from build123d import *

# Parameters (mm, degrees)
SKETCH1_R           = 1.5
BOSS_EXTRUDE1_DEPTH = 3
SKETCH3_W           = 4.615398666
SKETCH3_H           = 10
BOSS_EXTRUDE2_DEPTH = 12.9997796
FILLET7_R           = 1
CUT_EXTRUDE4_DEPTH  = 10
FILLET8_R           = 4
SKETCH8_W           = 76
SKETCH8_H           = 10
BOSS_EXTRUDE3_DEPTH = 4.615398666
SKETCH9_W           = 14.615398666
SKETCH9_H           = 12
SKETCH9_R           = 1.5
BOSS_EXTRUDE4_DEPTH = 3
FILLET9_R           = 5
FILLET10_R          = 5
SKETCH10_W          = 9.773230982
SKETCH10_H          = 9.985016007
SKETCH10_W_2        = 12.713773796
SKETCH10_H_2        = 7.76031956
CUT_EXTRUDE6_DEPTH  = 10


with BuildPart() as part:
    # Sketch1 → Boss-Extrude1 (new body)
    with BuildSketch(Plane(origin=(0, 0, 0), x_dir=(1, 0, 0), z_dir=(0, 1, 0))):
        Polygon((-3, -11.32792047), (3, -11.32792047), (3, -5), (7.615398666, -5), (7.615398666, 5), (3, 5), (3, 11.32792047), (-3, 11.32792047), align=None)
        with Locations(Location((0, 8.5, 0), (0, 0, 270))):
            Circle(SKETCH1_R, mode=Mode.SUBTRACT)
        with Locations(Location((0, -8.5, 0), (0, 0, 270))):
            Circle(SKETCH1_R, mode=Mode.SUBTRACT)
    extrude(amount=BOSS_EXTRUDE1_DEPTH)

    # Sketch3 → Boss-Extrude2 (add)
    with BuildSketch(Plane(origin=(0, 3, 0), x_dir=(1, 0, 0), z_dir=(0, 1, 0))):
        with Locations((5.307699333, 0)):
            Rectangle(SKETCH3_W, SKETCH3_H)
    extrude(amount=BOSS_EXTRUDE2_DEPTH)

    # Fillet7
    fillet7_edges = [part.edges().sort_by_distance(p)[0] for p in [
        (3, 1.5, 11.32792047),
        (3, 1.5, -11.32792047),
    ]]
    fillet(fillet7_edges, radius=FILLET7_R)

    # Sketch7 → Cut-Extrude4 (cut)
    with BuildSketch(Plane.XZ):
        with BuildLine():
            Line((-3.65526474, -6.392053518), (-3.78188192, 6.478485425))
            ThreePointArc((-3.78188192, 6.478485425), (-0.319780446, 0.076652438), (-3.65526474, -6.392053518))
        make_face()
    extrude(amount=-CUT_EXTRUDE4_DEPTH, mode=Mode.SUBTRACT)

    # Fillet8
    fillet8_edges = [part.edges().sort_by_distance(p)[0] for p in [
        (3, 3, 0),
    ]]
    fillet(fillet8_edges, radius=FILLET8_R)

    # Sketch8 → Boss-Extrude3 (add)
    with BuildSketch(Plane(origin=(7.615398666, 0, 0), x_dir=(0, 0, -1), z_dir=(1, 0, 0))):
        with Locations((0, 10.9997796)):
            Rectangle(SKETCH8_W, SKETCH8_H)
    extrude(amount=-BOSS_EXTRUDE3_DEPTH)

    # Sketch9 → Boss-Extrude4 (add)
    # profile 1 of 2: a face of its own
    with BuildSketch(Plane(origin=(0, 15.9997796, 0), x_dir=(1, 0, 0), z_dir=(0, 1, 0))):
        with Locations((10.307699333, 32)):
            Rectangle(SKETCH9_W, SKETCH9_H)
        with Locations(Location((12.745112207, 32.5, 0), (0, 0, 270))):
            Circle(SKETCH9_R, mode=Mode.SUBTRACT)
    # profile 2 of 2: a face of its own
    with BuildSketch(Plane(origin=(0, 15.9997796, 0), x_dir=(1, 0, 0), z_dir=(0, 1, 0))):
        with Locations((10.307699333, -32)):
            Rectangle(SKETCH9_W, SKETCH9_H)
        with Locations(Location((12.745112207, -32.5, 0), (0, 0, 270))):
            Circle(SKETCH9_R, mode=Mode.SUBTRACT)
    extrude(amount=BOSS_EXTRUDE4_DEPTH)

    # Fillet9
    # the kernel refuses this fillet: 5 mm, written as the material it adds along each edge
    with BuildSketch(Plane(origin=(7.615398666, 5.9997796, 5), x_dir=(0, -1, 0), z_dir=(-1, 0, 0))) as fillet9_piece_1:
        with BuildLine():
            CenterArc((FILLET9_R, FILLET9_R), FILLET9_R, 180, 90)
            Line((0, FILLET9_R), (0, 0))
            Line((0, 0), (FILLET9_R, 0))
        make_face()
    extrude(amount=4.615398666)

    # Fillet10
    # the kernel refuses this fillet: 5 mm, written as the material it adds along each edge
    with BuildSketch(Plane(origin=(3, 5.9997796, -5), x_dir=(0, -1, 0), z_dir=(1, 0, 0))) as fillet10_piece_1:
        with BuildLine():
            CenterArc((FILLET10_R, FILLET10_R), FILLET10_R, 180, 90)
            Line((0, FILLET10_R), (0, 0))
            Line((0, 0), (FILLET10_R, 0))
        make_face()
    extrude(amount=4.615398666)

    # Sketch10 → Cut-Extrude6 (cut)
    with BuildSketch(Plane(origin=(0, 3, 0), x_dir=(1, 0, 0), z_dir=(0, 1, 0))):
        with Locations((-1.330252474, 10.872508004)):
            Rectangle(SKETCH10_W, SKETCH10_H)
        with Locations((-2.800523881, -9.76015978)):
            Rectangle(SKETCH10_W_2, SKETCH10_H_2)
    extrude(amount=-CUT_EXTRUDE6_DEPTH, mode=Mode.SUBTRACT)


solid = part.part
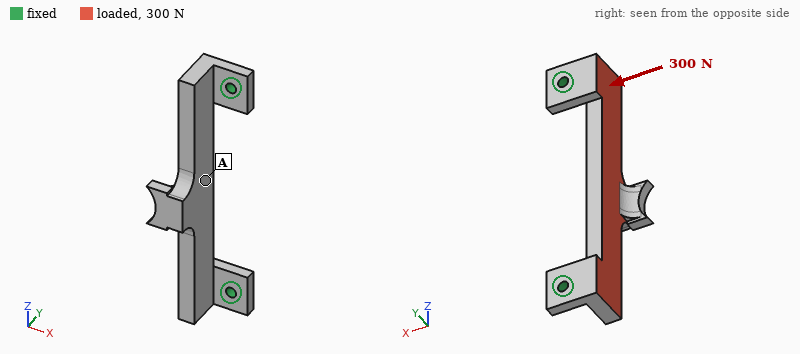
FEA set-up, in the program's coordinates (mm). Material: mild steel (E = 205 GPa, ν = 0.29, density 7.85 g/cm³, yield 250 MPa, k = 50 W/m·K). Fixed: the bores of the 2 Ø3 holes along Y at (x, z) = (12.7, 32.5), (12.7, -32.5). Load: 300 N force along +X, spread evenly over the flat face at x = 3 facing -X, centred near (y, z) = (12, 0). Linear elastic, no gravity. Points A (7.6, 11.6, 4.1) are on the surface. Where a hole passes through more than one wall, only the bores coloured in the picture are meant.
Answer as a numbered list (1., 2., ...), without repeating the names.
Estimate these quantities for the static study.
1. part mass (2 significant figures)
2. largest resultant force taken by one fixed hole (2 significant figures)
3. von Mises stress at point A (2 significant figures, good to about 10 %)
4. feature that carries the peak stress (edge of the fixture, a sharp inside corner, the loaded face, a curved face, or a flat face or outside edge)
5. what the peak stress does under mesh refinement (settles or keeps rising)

1. 39 g
2. 160 N
3. 13 MPa
4. edge of the fixture
5. keeps rising
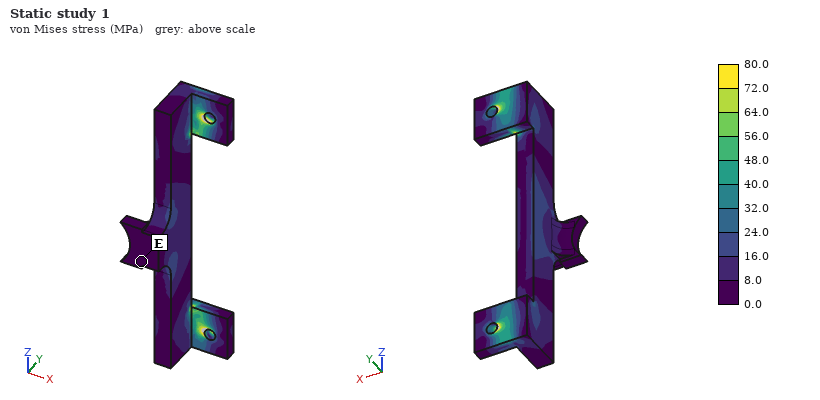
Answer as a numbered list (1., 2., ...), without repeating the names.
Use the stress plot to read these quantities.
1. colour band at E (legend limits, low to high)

1. 0.0 to 8.0 MPa
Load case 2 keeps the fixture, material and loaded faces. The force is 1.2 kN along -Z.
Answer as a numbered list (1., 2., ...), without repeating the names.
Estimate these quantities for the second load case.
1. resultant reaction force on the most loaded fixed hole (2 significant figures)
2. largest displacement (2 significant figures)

1. 610 N
2. 11 µm
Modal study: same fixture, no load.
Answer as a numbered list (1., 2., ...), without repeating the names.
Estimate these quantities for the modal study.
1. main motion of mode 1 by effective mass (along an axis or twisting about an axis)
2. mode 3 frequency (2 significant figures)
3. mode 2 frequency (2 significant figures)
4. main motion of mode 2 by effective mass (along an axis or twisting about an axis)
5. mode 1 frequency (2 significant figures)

1. along X
2. 8000 Hz
3. 6900 Hz
4. along Y
5. 3000 Hz
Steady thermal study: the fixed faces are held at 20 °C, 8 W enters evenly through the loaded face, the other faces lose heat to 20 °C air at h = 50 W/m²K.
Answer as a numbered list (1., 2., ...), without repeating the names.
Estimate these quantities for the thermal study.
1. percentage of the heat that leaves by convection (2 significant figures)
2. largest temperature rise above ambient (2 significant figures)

1. 26 %
2. 26 K
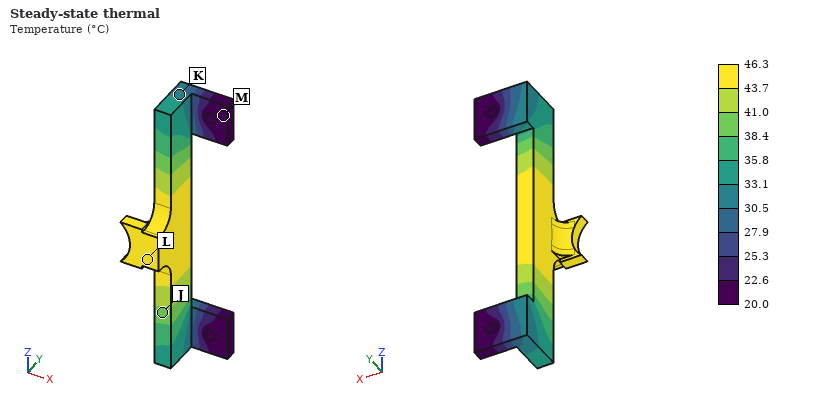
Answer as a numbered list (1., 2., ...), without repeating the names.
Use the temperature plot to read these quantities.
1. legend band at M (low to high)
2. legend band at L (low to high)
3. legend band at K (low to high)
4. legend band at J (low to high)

1. 20.0 to 22.6 °C
2. 43.7 to 46.3 °C
3. 30.5 to 33.1 °C
4. 38.4 to 41.0 °C
